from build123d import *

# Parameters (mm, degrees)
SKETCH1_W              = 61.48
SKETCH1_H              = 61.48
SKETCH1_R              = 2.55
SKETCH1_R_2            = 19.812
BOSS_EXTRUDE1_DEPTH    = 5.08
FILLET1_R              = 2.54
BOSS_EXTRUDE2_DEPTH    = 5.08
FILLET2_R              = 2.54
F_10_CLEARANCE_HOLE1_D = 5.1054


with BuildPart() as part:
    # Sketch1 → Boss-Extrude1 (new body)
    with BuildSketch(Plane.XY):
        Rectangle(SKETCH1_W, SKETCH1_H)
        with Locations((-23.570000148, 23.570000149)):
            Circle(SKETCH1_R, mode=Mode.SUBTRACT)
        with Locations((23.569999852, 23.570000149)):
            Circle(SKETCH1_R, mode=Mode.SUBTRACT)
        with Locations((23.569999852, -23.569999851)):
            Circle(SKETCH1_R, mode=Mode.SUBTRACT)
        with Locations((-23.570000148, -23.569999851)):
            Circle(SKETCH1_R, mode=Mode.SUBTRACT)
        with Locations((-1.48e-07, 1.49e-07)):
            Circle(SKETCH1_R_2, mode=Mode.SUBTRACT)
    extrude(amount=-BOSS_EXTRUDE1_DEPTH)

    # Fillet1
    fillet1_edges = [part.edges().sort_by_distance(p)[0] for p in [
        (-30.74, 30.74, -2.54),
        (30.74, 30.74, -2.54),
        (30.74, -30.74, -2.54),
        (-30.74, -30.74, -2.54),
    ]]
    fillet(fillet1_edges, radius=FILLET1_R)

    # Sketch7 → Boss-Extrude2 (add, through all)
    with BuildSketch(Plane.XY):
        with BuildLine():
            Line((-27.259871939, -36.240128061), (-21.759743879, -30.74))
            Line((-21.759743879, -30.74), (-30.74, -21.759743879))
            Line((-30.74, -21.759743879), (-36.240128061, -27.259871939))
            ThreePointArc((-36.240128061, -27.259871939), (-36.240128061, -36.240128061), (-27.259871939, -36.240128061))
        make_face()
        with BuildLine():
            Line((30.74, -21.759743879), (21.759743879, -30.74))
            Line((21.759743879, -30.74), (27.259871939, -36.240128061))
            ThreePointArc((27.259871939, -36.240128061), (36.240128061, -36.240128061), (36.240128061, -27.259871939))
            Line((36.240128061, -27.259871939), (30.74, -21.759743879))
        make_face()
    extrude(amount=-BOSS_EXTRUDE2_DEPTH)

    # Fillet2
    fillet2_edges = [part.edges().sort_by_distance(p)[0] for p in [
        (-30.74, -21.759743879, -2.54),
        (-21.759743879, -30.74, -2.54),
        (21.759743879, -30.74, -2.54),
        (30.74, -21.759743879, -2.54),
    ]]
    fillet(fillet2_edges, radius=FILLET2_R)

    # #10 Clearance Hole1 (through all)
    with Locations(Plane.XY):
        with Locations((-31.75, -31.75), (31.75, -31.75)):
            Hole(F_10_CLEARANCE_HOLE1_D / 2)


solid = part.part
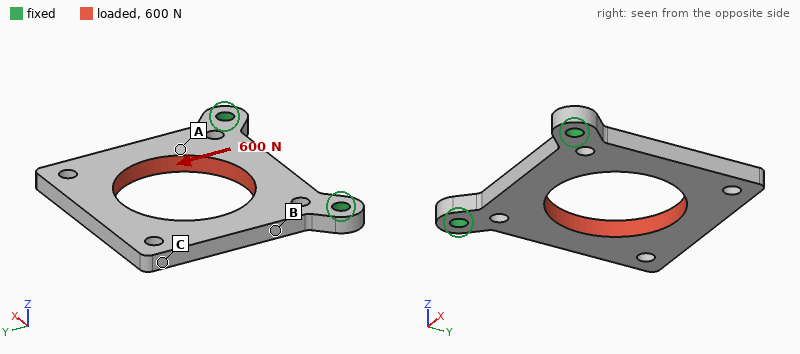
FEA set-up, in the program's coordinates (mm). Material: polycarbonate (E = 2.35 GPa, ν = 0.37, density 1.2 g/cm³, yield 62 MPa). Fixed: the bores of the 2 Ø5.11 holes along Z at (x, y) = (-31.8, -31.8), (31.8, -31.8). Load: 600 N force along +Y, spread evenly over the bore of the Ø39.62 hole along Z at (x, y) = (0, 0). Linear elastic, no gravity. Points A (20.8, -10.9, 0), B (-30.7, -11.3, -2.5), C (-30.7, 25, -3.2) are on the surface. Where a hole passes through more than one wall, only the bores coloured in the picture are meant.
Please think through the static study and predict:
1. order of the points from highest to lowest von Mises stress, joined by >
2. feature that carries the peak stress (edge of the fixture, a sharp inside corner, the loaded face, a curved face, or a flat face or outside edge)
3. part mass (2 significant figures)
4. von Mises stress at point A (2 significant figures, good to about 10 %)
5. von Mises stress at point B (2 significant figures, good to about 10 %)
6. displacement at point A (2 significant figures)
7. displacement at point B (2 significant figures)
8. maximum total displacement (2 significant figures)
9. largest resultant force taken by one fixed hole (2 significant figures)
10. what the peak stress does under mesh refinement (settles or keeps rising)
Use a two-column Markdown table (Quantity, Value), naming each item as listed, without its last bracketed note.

| Quantity | Value |
|---|---|
| order of the points from highest to lowest von Mises stress, joined by > | B > A > C |
| feature that carries the peak stress | edge of the fixture |
| part mass | 16 g |
| von Mises stress at point A | 2.5 MPa |
| von Mises stress at point B | 6.9 MPa |
| displacement at point A | 0.078 mm |
| displacement at point B | 0.067 mm |
| maximum total displacement | 0.12 mm |
| largest resultant force taken by one fixed hole | 330 N |
| what the peak stress does under mesh refinement | keeps rising |
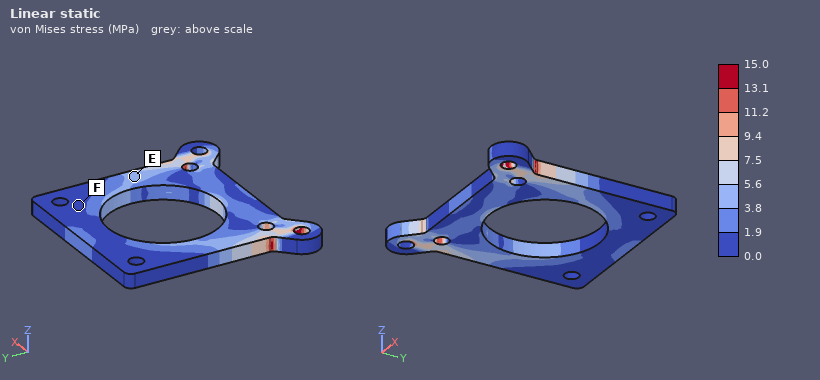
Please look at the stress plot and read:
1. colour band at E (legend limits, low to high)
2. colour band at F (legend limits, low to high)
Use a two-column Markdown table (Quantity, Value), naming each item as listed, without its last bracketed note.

| Quantity | Value |
|---|---|
| colour band at E | 3.8 to 5.6 MPa |
| colour band at F | 0.0 to 1.9 MPa |
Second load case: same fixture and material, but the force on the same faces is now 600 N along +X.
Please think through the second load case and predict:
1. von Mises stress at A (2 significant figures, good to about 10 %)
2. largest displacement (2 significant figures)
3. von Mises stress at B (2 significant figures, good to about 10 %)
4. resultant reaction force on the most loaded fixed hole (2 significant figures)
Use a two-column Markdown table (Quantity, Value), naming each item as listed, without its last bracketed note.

| Quantity | Value |
|---|---|
| von Mises stress at A | 6.5 MPa |
| largest displacement | 0.65 mm |
| von Mises stress at B | 11 MPa |
| resultant reaction force on the most loaded fixed hole | 410 N |
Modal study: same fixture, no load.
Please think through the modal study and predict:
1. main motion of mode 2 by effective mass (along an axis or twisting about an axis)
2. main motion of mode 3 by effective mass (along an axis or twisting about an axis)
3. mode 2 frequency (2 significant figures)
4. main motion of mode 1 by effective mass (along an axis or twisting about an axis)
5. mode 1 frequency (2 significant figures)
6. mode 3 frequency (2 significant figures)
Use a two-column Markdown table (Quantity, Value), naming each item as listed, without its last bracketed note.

| Quantity | Value |
|---|---|
| main motion of mode 2 by effective mass | twisting about Y |
| main motion of mode 3 by effective mass | along X |
| mode 2 frequency | 580 Hz |
| main motion of mode 1 by effective mass | along Z |
| mode 1 frequency | 210 Hz |
| mode 3 frequency | 1400 Hz |
